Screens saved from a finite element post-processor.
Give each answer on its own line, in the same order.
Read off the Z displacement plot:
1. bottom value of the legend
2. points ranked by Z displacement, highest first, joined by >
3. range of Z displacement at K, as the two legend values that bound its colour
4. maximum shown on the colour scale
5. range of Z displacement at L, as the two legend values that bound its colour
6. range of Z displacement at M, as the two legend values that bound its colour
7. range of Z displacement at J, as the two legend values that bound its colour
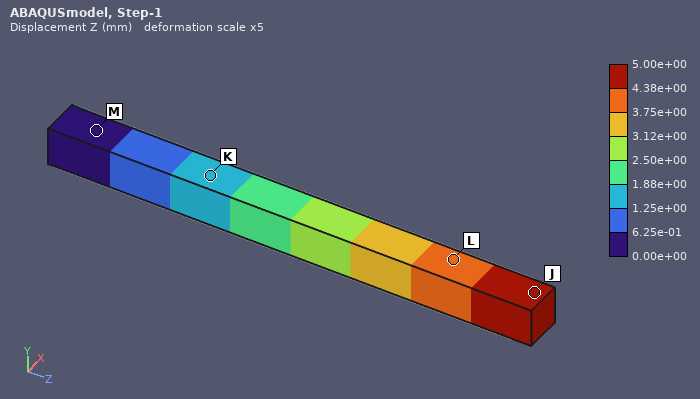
0.00e+00 mm
J > L > K > M
1.25e+00 to 1.88e+00 mm
5.00e+00 mm
3.75e+00 to 4.38e+00 mm
0.00e+00 to 6.25e-01 mm
4.38e+00 to 5.00e+00 mm
